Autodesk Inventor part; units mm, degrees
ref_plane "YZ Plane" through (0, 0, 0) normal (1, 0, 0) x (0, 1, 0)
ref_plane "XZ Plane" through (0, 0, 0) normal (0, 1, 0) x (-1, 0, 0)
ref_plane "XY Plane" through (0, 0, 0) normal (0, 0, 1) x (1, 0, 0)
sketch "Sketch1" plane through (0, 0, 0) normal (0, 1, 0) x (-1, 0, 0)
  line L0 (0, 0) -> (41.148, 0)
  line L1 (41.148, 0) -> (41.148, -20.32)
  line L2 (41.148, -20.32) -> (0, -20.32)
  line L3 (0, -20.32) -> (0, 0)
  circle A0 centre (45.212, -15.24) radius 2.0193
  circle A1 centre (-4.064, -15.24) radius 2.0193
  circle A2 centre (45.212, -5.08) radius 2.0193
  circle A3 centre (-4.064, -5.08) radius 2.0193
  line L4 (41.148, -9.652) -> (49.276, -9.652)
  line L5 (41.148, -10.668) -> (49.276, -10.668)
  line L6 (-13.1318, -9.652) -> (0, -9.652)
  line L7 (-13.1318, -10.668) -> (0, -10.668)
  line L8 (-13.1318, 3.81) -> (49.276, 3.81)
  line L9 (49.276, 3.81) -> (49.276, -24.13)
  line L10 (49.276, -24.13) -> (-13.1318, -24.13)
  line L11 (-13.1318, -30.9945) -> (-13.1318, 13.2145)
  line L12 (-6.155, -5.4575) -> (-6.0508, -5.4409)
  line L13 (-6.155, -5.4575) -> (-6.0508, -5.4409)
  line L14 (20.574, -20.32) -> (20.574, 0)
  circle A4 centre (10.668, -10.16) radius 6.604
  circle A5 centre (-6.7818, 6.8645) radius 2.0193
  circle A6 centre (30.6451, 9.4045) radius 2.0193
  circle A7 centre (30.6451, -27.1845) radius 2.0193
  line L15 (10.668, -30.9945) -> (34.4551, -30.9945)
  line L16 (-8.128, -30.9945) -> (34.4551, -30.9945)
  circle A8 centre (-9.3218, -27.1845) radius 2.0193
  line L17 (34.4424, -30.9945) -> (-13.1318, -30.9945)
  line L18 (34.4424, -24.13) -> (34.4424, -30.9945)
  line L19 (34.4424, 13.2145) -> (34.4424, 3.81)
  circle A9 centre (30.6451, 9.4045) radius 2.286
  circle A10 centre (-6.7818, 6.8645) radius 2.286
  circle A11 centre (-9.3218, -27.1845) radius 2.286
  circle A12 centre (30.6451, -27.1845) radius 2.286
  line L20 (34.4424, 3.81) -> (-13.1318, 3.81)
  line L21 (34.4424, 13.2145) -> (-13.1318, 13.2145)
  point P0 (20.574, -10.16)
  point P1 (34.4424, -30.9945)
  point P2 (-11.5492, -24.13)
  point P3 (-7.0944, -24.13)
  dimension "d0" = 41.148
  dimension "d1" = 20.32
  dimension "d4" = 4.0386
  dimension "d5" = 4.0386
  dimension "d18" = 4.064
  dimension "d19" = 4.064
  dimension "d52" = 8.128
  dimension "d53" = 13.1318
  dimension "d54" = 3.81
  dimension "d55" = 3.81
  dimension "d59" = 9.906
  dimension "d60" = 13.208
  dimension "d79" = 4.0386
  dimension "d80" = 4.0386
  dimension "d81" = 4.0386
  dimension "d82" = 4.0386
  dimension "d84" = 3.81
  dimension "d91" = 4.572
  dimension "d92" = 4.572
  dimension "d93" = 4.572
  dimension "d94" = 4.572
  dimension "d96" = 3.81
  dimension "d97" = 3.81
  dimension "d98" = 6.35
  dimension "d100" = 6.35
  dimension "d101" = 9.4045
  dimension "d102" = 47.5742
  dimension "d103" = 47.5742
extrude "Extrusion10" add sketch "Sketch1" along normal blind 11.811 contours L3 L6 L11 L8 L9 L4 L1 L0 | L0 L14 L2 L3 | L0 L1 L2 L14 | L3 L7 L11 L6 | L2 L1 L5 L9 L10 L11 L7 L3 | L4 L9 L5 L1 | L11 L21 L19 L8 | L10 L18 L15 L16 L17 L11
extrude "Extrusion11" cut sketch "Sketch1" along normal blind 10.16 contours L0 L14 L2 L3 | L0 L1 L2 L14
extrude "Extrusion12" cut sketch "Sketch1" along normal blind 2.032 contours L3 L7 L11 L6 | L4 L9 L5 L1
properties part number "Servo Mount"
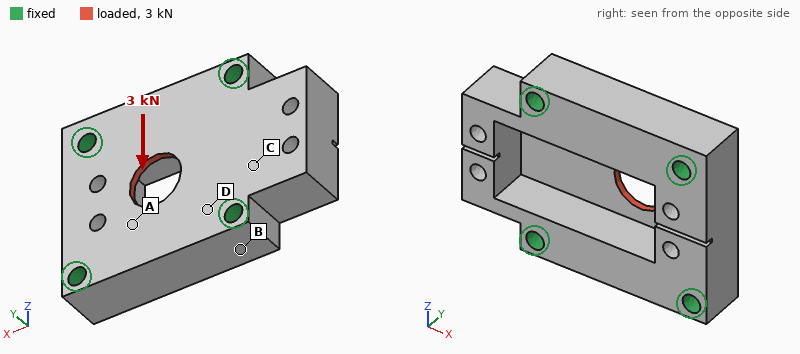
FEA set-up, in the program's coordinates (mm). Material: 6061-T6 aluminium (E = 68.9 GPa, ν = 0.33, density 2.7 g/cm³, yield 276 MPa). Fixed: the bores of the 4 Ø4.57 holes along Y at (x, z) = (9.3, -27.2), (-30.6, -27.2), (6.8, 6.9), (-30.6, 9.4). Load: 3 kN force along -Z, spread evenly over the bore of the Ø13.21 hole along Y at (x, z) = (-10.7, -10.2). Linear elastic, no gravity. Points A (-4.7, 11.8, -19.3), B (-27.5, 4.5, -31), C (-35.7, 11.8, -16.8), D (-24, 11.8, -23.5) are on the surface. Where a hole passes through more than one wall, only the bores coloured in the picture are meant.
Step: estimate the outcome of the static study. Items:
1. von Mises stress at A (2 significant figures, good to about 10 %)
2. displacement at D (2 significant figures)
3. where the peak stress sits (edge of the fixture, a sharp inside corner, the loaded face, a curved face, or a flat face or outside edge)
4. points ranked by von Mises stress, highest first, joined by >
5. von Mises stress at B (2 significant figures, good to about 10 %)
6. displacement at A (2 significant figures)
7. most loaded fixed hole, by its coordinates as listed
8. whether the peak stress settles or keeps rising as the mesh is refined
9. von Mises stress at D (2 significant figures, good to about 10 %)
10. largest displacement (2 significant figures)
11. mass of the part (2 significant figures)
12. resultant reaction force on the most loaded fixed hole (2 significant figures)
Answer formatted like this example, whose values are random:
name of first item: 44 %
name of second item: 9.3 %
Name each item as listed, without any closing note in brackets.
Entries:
von Mises stress at A: 36 MPa
displacement at D: 3.2 µm
where the peak stress sits: a sharp inside corner
points ranked by von Mises stress, highest first, joined by >: A > D > B > C
von Mises stress at B: 13 MPa
displacement at A: 7.2 µm
most loaded fixed hole, by its coordinates as listed: (6.8, 6.9)
whether the peak stress settles or keeps rising as the mesh is refined: keeps rising
von Mises stress at D: 24 MPa
largest displacement: 13 µm
mass of the part: 53 g
resultant reaction force on the most loaded fixed hole: 1.1 kN
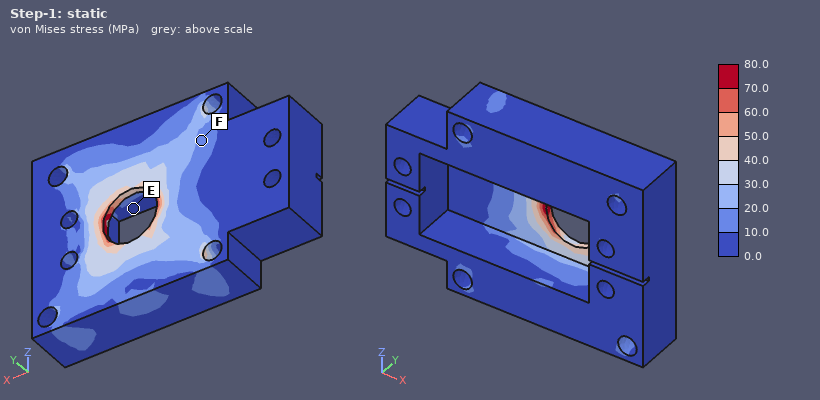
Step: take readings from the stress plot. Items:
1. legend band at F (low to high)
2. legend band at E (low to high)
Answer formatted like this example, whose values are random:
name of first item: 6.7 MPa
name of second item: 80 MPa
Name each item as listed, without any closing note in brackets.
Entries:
legend band at F: 10.0 to 20.0 MPa
legend band at E: 0.0 to 10.0 MPa
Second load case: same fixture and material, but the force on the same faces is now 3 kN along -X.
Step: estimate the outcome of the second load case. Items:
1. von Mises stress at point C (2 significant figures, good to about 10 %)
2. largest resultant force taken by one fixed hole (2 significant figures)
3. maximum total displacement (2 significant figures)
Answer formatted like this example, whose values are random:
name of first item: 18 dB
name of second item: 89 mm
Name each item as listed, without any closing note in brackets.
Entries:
von Mises stress at point C: 9.7 MPa
largest resultant force taken by one fixed hole: 910 N
maximum total displacement: 10 µm
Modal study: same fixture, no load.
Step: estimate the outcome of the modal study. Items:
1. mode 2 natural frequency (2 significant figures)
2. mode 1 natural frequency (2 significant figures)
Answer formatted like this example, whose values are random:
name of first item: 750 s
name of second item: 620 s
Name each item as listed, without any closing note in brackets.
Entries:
mode 2 natural frequency: 17 kHz
mode 1 natural frequency: 12 kHz
